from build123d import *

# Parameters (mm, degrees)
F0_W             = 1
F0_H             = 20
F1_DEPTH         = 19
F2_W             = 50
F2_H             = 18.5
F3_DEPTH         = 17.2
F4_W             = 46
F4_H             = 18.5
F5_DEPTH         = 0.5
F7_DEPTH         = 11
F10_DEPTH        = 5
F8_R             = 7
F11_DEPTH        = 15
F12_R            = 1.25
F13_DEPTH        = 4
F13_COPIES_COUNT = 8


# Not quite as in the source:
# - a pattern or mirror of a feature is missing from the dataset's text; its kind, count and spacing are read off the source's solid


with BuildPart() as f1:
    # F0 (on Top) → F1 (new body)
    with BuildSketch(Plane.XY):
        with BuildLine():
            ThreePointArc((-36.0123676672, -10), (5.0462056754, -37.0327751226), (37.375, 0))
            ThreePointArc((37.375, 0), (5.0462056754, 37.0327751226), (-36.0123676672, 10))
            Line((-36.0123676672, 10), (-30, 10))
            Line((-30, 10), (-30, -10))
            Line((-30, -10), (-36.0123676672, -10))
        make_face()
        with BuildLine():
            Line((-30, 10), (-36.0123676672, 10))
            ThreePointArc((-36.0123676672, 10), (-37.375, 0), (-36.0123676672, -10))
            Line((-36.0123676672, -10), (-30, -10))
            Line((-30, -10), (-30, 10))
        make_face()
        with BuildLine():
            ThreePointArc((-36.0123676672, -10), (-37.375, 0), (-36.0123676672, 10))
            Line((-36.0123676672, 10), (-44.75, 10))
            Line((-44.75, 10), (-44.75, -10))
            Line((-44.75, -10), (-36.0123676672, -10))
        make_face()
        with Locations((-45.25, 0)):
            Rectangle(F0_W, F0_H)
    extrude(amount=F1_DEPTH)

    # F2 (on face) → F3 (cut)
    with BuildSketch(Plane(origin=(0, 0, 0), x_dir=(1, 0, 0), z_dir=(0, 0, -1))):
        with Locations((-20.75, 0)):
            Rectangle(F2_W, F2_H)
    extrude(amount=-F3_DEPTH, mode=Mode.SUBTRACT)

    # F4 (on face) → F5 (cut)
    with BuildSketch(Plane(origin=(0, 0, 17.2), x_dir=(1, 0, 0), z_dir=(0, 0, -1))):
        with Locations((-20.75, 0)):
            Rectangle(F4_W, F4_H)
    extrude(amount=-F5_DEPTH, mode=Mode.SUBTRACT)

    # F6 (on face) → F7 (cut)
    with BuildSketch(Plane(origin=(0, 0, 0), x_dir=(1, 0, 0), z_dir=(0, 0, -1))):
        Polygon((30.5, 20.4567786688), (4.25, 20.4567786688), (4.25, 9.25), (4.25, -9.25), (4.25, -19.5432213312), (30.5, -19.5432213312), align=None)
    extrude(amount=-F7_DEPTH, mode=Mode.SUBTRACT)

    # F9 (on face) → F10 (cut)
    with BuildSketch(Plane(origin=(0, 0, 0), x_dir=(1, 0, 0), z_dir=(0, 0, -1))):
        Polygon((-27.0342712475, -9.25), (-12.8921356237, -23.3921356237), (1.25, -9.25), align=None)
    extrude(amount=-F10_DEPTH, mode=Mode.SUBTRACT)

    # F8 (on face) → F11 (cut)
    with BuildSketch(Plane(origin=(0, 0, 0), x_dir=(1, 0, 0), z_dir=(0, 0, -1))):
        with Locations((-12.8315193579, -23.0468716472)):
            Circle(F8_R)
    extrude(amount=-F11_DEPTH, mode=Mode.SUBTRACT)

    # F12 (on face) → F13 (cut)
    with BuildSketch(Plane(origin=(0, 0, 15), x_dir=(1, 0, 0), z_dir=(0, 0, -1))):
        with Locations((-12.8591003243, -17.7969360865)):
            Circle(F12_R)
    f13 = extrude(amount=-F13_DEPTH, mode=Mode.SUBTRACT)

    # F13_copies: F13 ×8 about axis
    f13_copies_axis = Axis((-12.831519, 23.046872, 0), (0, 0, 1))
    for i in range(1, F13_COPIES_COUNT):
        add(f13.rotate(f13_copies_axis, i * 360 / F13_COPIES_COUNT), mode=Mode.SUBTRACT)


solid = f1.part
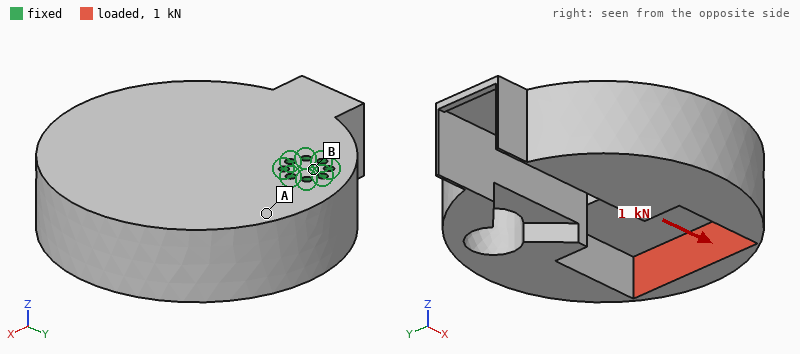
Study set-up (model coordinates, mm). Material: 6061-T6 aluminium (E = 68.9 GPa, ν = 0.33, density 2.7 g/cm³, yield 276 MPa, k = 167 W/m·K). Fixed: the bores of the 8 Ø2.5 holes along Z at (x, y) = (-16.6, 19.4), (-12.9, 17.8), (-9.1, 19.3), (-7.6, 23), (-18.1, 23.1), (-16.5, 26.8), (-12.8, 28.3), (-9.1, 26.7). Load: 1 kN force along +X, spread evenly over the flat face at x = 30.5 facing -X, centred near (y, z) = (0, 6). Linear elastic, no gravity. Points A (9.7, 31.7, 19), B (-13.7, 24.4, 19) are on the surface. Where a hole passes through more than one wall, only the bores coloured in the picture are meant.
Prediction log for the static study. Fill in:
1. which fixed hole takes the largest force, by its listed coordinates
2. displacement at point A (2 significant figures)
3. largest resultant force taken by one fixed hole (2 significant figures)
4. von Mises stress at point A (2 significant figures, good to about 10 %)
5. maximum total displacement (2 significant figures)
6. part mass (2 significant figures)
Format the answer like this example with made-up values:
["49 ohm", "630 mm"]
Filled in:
["(-12.9, 17.8)", "0.017 mm", "770 N", "11 MPa", "0.10 mm", "150 g"]
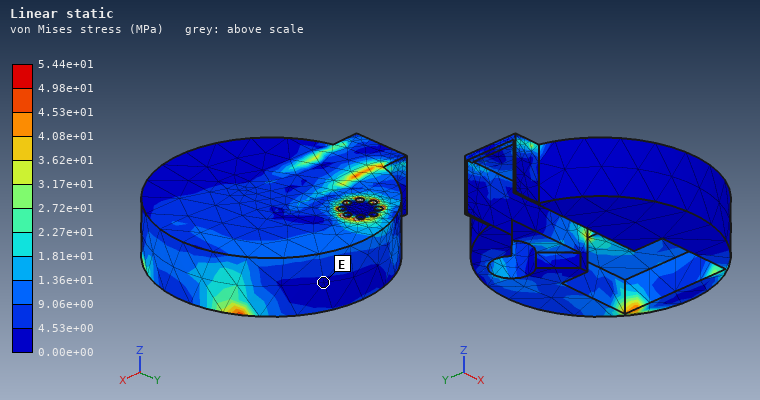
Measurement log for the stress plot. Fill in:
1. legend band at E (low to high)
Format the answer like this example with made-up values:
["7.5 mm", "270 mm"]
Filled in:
["0.00e+00 to 4.53e+00 MPa"]
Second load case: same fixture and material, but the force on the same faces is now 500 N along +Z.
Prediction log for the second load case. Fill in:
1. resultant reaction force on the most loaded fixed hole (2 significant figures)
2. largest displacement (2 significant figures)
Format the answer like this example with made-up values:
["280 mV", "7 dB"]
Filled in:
["810 N", "0.14 mm"]
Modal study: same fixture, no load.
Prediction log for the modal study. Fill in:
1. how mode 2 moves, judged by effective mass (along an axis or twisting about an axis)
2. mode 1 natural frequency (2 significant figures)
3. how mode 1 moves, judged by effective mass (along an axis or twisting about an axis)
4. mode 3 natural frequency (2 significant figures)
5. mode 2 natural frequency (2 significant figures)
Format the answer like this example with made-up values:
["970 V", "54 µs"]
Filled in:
["along X", "990 Hz", "along Z", "2500 Hz", "1600 Hz"]
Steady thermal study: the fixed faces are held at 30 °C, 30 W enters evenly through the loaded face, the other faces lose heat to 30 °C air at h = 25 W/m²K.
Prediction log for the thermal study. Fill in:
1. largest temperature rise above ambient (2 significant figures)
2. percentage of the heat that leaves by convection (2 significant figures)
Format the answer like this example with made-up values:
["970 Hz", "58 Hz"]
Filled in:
["27 K", "16 %"]
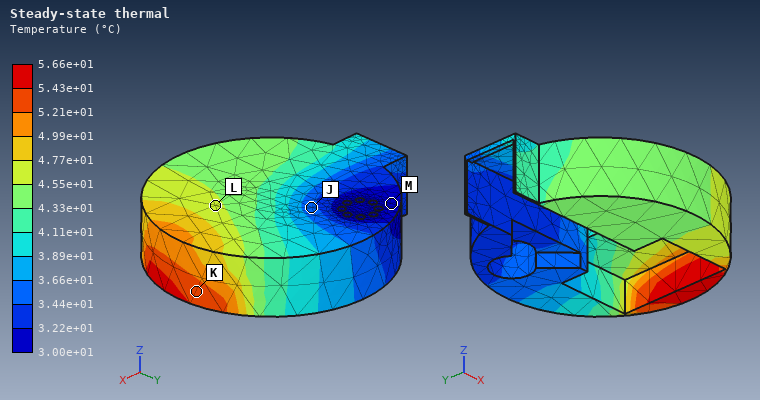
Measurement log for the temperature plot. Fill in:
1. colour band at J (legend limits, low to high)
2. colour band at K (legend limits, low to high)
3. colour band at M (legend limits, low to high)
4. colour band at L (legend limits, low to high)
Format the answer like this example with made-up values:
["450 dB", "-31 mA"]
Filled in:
["3.44e+01 to 3.66e+01 °C", "5.21e+01 to 5.43e+01 °C", "3.00e+01 to 3.22e+01 °C", "4.55e+01 to 4.77e+01 °C"]
